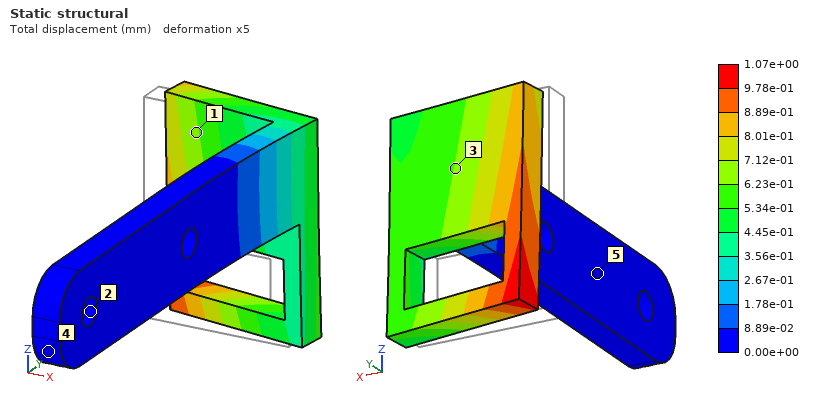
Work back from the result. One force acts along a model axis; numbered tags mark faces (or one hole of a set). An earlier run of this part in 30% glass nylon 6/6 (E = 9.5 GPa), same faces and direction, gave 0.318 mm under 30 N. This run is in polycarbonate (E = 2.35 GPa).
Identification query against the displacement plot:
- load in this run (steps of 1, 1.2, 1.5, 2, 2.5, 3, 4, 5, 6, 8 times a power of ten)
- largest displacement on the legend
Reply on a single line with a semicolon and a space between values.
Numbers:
25 N; 1.07e+00 mm
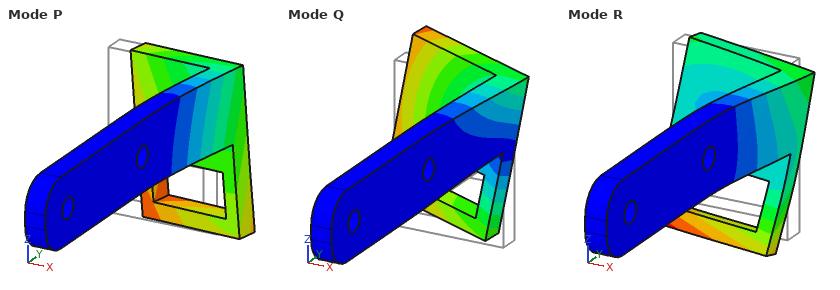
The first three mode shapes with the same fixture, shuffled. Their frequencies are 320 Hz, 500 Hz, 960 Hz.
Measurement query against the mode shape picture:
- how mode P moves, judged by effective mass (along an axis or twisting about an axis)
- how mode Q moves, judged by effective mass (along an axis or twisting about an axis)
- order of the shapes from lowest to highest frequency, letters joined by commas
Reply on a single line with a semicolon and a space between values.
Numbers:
along X; along Z; P, Q, R
